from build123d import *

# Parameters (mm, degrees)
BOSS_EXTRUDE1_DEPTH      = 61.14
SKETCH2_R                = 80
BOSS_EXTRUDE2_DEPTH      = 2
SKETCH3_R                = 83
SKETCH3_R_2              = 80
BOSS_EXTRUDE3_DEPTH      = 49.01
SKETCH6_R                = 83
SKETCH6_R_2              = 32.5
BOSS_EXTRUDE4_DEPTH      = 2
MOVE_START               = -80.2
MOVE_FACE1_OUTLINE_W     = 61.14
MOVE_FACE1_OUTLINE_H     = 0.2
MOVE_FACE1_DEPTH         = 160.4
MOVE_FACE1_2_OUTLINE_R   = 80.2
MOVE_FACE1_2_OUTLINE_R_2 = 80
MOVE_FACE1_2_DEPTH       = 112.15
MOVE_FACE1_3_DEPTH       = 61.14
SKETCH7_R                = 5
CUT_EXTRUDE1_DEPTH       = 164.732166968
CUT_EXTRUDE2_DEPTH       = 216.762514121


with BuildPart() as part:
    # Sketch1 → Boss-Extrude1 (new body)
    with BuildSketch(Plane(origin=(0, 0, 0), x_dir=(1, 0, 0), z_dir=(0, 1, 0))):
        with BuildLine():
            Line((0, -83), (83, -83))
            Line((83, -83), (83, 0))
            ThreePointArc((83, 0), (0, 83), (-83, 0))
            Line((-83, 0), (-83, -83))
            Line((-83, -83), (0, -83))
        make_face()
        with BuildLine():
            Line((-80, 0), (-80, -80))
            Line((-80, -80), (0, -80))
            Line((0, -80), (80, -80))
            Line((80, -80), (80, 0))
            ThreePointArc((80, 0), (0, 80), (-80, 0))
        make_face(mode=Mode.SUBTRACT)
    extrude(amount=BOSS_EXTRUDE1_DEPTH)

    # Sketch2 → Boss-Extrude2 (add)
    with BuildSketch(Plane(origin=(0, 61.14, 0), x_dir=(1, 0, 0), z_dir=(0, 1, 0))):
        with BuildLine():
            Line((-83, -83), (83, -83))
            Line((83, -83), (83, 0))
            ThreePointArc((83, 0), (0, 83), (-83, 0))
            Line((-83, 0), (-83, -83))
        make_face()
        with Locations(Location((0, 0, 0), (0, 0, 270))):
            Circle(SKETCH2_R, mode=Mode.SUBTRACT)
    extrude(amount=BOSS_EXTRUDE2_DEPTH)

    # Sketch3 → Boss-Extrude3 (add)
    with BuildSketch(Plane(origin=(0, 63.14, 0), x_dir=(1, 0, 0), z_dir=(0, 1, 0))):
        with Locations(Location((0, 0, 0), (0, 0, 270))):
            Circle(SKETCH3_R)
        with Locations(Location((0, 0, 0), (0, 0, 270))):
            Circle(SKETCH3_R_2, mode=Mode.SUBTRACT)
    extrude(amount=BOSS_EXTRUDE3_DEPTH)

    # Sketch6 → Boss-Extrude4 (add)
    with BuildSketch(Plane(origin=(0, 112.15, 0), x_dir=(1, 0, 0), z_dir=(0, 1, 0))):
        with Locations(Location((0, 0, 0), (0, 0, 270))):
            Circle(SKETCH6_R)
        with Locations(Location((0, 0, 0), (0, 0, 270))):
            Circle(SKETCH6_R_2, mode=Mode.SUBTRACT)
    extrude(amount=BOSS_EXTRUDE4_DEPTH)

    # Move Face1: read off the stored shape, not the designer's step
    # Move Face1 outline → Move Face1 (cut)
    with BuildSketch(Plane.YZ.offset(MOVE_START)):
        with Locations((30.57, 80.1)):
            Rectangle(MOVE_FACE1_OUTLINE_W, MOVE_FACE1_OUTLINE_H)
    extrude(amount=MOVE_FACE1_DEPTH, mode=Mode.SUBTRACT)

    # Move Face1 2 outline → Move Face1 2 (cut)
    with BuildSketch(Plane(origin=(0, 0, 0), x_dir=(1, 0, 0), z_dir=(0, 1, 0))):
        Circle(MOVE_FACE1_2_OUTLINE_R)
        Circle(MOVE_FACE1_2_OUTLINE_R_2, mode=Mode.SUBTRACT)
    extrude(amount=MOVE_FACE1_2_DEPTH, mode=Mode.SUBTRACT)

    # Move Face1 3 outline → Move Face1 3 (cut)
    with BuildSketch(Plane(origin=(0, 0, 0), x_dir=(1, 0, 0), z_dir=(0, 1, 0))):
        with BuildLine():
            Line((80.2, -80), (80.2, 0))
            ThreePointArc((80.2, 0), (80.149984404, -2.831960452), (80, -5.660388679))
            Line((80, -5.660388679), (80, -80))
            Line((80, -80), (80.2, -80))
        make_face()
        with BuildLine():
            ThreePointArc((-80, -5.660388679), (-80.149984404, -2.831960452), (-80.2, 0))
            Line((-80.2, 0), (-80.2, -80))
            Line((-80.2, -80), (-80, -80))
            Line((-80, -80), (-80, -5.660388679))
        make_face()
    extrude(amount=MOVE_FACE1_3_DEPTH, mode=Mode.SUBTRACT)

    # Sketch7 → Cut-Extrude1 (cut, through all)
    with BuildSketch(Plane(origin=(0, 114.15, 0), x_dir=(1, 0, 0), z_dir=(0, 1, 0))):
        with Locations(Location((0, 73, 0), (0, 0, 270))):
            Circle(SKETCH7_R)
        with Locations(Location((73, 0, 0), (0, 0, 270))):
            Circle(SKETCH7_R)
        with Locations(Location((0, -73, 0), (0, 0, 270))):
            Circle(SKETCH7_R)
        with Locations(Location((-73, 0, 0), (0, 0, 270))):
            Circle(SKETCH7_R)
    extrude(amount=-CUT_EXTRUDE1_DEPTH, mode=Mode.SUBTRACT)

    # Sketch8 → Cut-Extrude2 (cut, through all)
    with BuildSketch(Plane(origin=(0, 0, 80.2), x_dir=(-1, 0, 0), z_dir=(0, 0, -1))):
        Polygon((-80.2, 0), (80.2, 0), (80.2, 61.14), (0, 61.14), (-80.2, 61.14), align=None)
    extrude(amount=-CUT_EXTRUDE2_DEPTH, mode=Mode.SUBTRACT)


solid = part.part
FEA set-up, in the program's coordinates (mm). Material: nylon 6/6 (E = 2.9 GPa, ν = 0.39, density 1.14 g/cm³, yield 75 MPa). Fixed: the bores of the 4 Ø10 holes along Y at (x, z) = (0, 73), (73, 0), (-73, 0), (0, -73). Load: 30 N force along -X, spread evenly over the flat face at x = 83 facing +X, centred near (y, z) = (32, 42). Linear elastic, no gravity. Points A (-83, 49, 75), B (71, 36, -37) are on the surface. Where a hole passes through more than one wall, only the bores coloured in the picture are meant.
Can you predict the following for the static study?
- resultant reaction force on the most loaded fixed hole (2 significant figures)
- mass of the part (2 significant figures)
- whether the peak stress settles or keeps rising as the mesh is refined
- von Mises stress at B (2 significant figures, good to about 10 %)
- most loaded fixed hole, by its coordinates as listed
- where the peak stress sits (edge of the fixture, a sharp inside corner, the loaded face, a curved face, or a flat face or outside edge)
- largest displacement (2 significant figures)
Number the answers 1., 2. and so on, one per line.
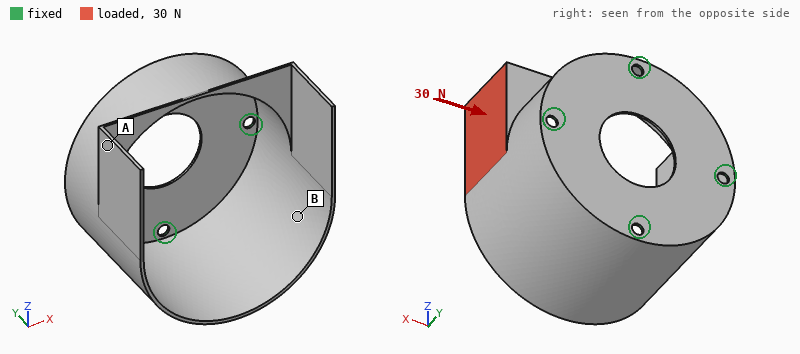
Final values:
1. 41 N
2. 210 g
3. keeps rising
4. 1.4 MPa
5. (73, 0)
6. edge of the fixture
7. 2.5 mm
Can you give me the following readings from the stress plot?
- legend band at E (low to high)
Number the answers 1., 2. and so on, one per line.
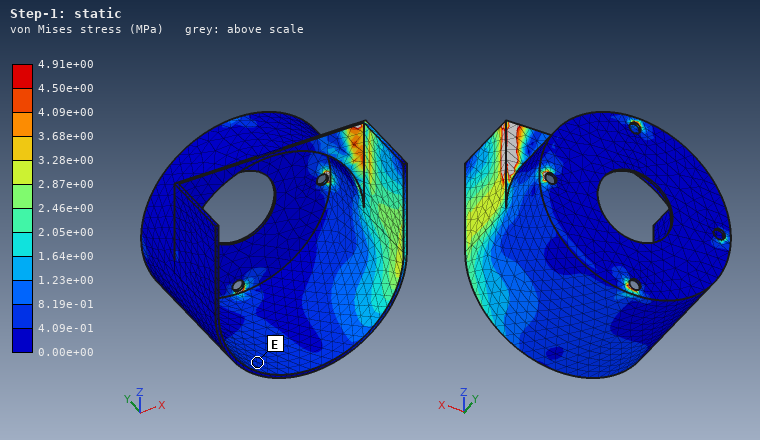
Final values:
1. 4.09e-01 to 8.19e-01 MPa
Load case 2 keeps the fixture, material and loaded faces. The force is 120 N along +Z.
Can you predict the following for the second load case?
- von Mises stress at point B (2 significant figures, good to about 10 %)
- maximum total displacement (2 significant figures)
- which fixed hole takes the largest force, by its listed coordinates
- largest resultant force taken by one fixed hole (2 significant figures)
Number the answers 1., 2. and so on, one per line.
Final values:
1. 4.0 MPa
2. 2.5 mm
3. (73, 0)
4. 89 N
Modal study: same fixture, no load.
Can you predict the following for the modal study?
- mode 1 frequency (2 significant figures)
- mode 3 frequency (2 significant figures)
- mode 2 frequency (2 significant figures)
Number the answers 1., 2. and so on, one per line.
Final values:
1. 120 Hz
2. 200 Hz
3. 190 Hz
